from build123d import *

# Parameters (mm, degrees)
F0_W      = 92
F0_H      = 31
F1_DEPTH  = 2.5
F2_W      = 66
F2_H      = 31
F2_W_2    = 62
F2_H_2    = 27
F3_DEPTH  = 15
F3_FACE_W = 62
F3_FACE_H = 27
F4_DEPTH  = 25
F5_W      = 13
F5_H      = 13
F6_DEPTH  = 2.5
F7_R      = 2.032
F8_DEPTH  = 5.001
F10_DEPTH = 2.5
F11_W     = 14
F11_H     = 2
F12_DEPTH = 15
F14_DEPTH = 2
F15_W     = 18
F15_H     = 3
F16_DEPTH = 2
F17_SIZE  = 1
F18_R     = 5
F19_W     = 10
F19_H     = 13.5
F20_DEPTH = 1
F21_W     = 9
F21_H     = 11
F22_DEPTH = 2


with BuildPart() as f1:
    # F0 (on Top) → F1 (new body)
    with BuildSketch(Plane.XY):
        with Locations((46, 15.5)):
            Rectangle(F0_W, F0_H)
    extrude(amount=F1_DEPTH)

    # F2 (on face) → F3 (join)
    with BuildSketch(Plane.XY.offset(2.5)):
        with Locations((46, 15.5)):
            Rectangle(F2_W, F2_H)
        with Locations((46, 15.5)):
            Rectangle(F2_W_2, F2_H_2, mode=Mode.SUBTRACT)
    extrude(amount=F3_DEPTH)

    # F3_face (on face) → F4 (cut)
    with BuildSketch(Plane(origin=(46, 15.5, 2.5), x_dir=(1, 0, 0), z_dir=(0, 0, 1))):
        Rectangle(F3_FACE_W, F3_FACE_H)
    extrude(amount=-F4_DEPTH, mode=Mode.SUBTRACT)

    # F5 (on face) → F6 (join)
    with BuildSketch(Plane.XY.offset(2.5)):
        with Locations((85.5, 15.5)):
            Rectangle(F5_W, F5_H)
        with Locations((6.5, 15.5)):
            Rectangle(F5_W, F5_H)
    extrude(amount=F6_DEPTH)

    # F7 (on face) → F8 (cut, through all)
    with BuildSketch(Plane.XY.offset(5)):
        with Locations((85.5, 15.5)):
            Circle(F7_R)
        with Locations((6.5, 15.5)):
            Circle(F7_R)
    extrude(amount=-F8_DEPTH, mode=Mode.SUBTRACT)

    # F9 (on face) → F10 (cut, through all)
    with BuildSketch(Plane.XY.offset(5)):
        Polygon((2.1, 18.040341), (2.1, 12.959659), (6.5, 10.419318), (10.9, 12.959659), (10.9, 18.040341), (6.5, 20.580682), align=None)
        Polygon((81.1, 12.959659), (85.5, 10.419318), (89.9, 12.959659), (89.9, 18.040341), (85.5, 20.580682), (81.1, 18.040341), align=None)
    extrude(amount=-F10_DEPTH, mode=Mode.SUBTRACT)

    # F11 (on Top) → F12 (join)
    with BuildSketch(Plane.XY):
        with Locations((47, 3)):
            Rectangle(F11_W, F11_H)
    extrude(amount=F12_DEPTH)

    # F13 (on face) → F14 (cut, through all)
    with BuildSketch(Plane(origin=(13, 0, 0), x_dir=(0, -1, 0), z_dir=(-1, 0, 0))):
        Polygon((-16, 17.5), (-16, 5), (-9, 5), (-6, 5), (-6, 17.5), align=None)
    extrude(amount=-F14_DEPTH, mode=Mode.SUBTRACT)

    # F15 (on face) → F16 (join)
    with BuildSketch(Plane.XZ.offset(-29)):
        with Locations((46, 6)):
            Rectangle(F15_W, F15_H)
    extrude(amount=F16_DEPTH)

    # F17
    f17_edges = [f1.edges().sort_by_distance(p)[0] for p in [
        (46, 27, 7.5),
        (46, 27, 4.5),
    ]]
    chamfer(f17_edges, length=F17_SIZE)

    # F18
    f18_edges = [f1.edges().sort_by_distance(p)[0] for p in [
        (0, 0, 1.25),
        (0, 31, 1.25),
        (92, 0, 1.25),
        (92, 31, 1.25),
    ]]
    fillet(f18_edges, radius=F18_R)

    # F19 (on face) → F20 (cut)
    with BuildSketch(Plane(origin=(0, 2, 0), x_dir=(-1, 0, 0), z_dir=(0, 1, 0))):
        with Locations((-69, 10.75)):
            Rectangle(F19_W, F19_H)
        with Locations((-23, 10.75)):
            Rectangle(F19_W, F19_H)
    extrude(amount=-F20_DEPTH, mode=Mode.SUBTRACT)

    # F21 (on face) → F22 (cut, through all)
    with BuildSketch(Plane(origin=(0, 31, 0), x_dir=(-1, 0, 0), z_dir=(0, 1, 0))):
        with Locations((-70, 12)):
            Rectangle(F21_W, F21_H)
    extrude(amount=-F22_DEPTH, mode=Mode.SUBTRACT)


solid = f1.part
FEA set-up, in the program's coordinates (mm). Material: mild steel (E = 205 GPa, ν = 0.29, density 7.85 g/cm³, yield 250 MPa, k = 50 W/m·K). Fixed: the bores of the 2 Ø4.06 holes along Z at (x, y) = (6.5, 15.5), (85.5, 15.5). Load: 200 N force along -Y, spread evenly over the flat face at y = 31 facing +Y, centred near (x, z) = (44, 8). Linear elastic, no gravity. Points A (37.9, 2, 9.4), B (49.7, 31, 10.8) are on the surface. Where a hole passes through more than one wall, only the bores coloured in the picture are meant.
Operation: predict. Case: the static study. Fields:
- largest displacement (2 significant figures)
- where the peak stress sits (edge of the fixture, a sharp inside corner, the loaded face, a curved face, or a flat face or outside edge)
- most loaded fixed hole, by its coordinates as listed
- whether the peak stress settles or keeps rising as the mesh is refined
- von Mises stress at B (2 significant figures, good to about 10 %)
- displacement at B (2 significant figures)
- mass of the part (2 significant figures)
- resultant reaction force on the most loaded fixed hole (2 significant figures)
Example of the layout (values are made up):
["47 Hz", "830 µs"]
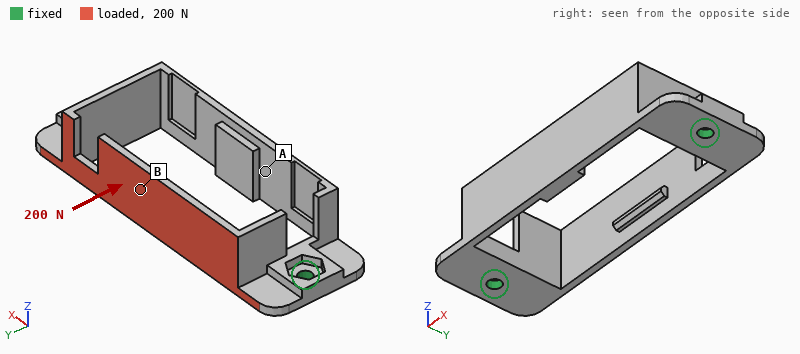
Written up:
["94 µm", "a sharp inside corner", "(6.5, 15.5)", "keeps rising", "37 MPa", "78 µm", "68 g", "120 N"]
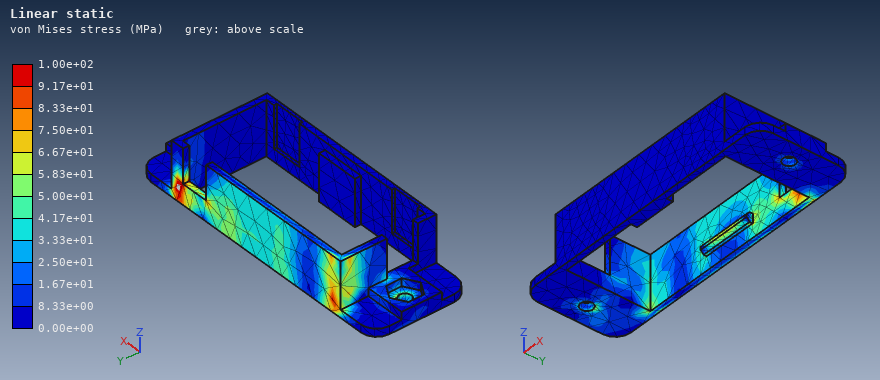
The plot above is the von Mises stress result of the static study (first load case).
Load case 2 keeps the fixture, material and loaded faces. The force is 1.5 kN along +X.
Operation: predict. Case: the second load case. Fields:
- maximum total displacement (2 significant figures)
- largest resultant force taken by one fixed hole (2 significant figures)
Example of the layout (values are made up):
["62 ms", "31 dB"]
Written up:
["42 µm", "770 N"]
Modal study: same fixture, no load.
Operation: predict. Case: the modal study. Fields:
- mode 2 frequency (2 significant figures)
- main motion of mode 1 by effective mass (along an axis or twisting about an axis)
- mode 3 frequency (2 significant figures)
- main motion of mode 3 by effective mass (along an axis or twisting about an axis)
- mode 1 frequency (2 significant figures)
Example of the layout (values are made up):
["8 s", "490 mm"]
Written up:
["2100 Hz", "along Y", "3200 Hz", "twisting about X", "1900 Hz"]
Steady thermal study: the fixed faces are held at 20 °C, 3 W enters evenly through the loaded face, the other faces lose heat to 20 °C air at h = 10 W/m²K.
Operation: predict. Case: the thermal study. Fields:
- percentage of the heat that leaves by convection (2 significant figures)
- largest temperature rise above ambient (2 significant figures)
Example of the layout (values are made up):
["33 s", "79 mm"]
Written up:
["16 %", "27 K"]
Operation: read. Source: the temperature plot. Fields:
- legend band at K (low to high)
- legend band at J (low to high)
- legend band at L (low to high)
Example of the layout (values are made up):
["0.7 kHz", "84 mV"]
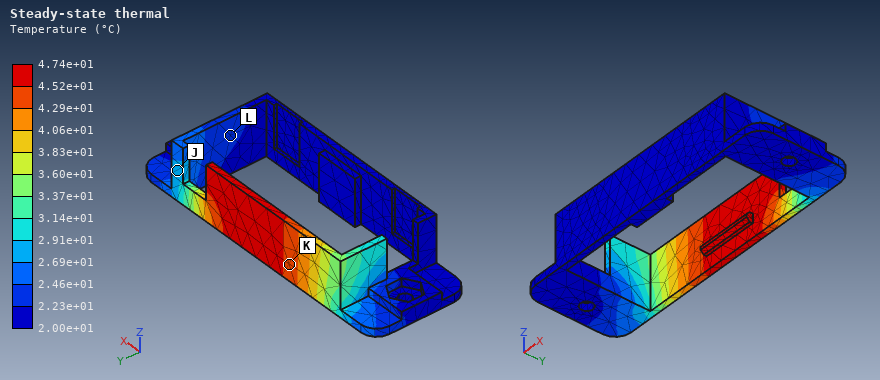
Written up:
["4.29e+01 to 4.52e+01 °C", "2.69e+01 to 2.91e+01 °C", "2.23e+01 to 2.46e+01 °C"]
